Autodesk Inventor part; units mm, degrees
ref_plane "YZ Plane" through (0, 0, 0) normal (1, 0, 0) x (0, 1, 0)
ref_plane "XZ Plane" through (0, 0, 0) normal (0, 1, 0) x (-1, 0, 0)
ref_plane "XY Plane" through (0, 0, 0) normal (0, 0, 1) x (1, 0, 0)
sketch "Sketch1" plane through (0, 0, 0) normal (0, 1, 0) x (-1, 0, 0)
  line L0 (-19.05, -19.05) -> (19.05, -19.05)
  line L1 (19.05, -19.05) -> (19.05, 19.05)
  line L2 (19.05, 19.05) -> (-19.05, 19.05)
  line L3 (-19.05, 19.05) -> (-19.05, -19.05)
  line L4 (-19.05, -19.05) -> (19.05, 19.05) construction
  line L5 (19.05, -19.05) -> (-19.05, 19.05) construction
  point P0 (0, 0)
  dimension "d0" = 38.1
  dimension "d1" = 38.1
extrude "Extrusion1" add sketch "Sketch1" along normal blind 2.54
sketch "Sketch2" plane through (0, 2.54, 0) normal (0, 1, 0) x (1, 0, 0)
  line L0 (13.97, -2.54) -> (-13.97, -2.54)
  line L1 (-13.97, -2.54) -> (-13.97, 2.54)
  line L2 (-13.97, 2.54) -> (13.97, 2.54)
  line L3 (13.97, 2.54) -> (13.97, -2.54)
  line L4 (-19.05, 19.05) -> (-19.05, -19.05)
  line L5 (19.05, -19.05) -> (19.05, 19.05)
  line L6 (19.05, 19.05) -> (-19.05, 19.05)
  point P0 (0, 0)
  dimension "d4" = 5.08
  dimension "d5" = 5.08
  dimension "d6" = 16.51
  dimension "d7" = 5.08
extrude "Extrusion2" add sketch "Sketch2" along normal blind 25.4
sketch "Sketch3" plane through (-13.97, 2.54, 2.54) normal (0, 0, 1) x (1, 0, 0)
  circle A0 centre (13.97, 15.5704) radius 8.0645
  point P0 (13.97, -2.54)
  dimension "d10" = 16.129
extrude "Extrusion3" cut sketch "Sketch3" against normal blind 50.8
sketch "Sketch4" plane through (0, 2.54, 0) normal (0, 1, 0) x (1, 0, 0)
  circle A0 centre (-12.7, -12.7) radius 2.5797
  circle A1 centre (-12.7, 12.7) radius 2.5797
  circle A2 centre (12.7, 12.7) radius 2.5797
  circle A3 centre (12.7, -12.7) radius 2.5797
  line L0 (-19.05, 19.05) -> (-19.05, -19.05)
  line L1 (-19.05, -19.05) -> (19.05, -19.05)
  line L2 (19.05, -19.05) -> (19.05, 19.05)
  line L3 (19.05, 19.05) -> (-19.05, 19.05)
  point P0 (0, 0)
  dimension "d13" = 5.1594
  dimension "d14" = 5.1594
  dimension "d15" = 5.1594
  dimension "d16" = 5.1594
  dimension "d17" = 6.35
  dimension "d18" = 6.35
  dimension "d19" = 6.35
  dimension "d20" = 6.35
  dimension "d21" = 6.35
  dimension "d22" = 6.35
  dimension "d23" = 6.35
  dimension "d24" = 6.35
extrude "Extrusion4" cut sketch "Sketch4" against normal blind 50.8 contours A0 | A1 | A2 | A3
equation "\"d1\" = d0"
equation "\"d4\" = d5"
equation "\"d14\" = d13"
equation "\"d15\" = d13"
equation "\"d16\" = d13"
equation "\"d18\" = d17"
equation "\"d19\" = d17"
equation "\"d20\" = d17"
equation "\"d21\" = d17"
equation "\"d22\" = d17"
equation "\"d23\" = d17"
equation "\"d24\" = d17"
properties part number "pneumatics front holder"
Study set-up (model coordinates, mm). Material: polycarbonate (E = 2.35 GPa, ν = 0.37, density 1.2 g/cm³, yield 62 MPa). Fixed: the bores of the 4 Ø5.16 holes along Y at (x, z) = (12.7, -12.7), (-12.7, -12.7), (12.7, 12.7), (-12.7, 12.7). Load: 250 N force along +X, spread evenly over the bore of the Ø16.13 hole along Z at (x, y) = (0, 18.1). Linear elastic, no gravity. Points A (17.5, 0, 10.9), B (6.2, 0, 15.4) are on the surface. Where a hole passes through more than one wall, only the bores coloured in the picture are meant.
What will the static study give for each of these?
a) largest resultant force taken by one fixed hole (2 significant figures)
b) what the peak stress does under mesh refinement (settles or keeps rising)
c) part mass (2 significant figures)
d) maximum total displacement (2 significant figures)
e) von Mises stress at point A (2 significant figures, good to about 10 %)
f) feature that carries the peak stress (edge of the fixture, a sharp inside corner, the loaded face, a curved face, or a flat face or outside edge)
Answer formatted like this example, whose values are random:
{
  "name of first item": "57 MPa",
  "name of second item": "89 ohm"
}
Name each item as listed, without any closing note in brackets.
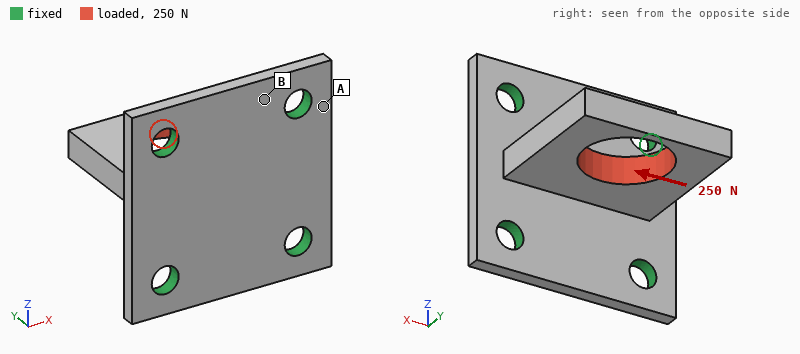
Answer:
{
  "largest resultant force taken by one fixed hole": "110 N",
  "what the peak stress does under mesh refinement": "keeps rising",
  "part mass": "7.3 g",
  "maximum total displacement": "0.68 mm",
  "von Mises stress at point A": "12 MPa",
  "feature that carries the peak stress": "edge of the fixture"
}
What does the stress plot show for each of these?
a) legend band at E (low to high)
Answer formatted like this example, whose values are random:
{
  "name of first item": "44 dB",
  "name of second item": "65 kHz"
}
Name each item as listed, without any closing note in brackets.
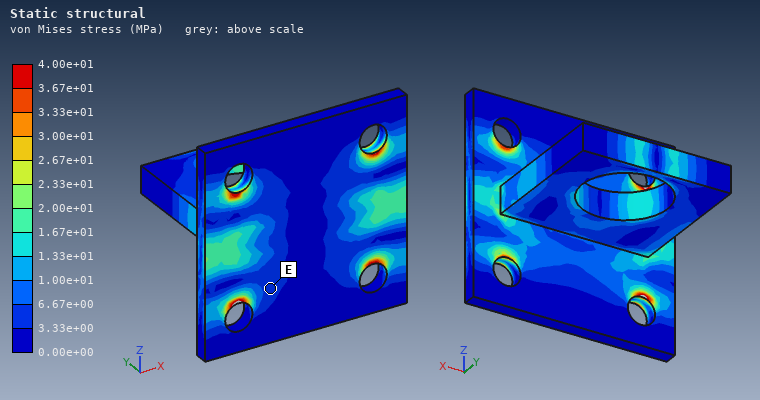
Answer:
{
  "legend band at E": "3.33e+00 to 6.67e+00 MPa"
}
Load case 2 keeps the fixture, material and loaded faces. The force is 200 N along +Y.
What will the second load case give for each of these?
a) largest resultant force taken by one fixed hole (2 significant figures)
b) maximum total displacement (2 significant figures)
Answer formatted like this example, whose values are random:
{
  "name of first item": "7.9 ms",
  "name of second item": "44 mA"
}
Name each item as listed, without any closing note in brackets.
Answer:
{
  "largest resultant force taken by one fixed hole": "51 N",
  "maximum total displacement": "0.16 mm"
}
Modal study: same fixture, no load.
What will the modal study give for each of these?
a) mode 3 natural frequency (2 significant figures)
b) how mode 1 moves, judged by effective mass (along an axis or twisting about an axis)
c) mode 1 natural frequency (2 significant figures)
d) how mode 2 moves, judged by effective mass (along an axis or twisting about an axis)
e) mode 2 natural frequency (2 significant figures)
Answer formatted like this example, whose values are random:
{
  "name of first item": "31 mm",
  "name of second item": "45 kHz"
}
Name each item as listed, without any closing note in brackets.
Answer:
{
  "mode 3 natural frequency": "2600 Hz",
  "how mode 1 moves, judged by effective mass": "along Z",
  "mode 1 natural frequency": "1300 Hz",
  "how mode 2 moves, judged by effective mass": "along X",
  "mode 2 natural frequency": "2300 Hz"
}
